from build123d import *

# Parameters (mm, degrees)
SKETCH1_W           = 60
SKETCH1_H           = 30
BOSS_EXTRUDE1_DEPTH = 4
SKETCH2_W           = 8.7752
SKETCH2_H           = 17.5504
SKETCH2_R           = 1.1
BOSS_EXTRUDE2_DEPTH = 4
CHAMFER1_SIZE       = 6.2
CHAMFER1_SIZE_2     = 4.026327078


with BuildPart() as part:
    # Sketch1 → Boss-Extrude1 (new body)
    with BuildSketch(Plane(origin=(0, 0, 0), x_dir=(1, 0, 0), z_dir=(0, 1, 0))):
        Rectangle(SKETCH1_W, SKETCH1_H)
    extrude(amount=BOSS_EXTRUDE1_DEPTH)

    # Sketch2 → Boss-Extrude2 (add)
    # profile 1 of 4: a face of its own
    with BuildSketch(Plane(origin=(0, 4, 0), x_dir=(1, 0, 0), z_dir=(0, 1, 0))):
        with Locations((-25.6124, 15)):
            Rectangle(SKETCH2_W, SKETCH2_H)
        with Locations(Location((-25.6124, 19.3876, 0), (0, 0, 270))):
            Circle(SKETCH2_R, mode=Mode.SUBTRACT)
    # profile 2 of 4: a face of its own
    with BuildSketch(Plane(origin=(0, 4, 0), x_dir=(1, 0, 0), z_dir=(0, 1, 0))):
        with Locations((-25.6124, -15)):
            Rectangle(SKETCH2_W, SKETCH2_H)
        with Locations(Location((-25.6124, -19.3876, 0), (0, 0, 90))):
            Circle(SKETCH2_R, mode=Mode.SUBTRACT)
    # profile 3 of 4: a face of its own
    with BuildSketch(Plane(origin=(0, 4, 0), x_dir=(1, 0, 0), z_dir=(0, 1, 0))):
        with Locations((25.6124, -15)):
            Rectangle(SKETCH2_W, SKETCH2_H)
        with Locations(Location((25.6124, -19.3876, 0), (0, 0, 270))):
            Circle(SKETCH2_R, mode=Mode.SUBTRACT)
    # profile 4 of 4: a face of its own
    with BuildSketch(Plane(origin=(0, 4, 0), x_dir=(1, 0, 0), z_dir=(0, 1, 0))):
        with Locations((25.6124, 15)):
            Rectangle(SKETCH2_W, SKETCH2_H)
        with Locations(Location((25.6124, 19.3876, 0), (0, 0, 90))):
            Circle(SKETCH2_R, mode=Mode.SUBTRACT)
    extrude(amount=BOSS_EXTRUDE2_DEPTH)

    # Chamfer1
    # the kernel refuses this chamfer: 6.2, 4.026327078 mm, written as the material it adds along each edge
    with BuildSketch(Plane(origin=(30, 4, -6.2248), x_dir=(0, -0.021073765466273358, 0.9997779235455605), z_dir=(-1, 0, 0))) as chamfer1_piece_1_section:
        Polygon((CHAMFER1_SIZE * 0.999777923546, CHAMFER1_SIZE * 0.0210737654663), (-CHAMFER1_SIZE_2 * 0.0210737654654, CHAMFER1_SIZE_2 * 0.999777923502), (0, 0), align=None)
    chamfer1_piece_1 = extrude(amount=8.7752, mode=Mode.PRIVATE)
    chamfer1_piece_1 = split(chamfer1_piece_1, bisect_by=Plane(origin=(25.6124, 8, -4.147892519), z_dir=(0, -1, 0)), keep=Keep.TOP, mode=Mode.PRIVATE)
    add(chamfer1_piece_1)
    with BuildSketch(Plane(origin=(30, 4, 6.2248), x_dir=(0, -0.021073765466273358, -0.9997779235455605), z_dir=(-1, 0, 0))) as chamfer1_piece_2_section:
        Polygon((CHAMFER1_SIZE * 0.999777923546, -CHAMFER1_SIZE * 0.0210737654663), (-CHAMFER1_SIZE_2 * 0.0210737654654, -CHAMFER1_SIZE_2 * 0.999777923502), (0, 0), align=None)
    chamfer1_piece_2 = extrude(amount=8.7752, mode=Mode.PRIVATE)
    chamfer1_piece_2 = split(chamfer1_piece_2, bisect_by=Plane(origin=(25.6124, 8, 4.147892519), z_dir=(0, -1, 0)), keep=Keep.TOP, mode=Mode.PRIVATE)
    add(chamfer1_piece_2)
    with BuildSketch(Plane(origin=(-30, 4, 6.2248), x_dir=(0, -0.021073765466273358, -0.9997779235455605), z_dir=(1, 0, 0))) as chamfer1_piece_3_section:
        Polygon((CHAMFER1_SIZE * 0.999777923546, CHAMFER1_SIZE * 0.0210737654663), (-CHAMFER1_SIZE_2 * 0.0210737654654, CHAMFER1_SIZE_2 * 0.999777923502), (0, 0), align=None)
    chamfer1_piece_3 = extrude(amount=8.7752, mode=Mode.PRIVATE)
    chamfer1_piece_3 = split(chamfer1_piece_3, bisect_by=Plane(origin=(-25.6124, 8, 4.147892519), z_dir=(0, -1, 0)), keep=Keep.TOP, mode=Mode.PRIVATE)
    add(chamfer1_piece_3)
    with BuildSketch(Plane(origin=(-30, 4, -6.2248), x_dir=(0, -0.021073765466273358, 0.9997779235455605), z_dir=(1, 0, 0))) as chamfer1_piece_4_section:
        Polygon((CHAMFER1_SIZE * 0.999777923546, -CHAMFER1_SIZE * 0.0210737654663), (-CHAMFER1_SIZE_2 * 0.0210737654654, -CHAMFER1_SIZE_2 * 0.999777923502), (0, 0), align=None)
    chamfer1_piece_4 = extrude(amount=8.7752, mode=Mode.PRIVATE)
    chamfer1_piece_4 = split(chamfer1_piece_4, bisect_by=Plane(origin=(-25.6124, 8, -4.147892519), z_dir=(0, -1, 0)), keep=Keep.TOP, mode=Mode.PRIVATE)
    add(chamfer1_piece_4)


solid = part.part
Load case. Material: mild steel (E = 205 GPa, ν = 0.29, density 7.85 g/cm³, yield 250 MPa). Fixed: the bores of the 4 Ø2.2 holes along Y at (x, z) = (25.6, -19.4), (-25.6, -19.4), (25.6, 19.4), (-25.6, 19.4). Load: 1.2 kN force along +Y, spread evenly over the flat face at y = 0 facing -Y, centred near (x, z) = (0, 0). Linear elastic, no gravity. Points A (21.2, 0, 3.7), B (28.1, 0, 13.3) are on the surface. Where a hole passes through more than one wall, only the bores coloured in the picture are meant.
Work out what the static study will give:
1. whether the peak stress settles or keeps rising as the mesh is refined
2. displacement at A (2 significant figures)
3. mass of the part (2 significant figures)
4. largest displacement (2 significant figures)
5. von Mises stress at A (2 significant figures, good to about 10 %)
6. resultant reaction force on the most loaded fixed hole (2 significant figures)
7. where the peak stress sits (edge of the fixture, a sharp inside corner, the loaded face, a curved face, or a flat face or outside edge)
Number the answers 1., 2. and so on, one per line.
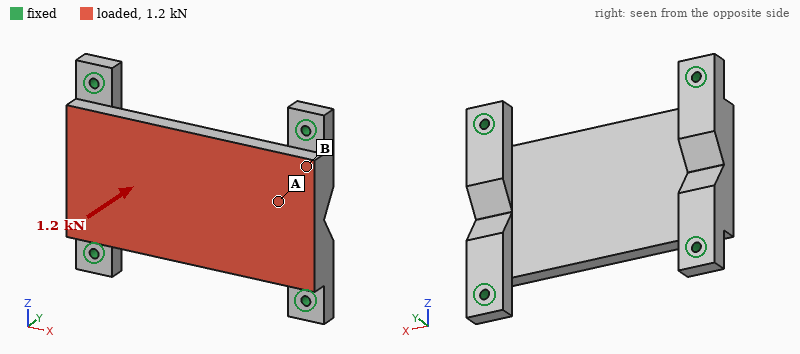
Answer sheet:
1. keeps rising
2. 5.9 µm
3. 79 g
4. 17 µm
5. 22 MPa
6. 560 N
7. edge of the fixture
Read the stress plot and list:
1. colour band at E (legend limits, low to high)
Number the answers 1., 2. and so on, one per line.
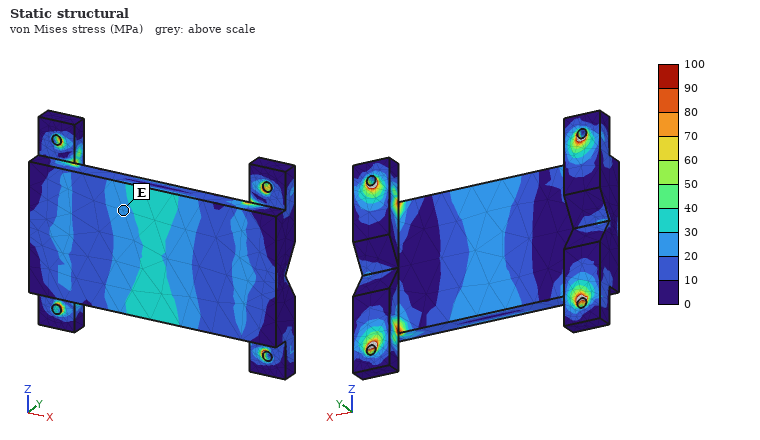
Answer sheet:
1. 20 to 30 MPa
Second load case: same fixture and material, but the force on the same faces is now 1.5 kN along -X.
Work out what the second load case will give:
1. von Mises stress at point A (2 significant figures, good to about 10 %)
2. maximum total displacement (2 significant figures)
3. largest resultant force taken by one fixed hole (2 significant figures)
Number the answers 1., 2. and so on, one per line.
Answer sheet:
1. 16 MPa
2. 5.3 µm
3. 400 N
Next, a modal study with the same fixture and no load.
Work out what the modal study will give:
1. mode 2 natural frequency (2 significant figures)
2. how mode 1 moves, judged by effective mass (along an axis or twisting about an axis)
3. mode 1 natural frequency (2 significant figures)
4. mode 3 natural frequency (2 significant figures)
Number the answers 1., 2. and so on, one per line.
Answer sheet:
1. 11 kHz
2. along Y
3. 6400 Hz
4. 11 kHz
